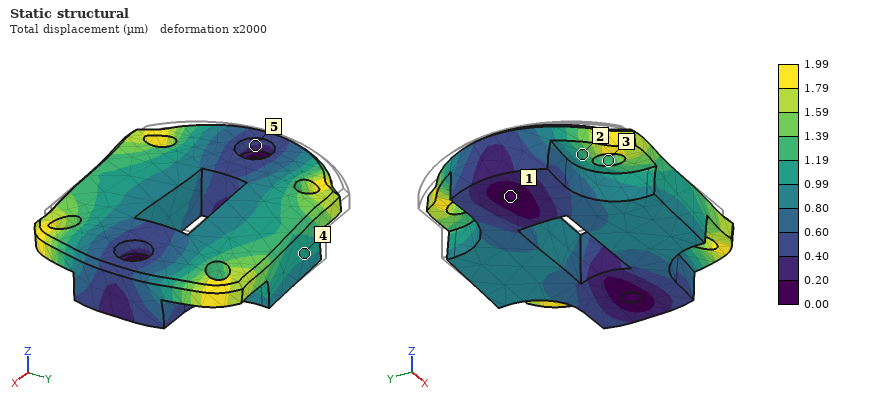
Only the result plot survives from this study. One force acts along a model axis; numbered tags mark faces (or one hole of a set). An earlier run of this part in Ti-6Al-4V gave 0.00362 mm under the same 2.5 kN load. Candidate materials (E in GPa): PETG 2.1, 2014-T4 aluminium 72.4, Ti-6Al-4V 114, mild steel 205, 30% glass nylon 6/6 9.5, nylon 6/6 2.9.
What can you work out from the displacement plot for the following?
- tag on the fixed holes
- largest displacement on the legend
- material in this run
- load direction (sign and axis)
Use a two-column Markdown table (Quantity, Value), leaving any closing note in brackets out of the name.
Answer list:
| Quantity | Value |
|---|---|
| tag on the fixed holes | 1 |
| largest displacement on the legend | 1.99 µm |
| material in this run | mild steel |
| load direction | +X |
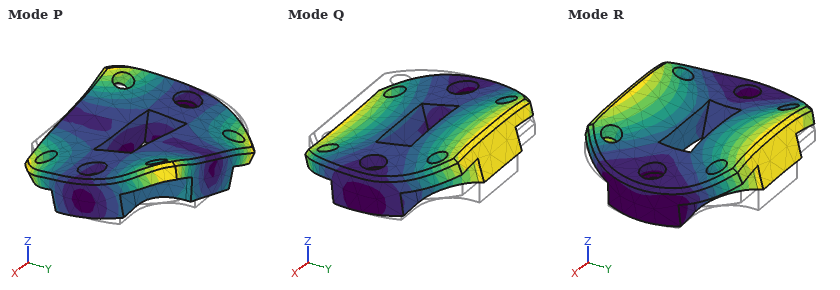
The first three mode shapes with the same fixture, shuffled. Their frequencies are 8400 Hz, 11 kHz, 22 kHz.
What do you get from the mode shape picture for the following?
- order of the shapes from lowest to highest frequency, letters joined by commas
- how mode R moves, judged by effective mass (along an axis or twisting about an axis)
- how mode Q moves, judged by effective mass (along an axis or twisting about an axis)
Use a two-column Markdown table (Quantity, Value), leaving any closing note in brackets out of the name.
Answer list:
| Quantity | Value |
|---|---|
| order of the shapes from lowest to highest frequency, letters joined by commas | Q, R, P |
| how mode R moves, judged by effective mass | along Z |
| how mode Q moves, judged by effective mass | twisting about X |
